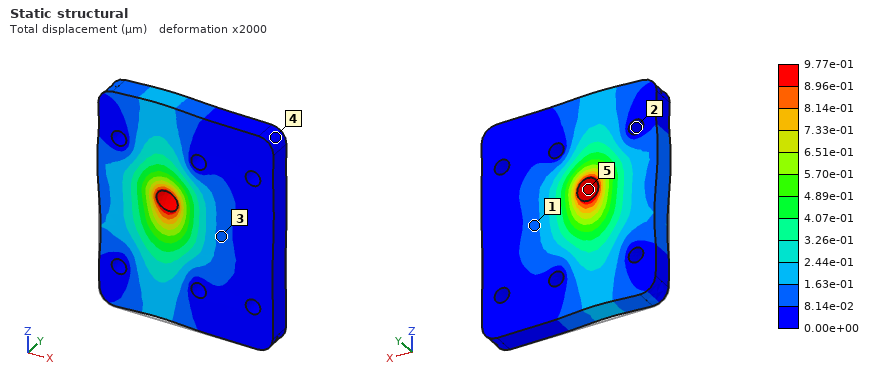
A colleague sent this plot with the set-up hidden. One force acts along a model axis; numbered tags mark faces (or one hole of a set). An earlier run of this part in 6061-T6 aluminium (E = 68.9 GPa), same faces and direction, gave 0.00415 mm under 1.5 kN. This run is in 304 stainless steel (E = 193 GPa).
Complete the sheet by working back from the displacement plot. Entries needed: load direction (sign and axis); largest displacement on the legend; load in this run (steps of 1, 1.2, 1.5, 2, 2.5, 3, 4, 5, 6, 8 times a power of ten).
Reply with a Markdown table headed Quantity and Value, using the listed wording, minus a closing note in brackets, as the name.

| Quantity | Value |
|---|---|
| load direction | +Z |
| largest displacement on the legend | 9.77e-01 µm |
| load in this run | 1 kN |
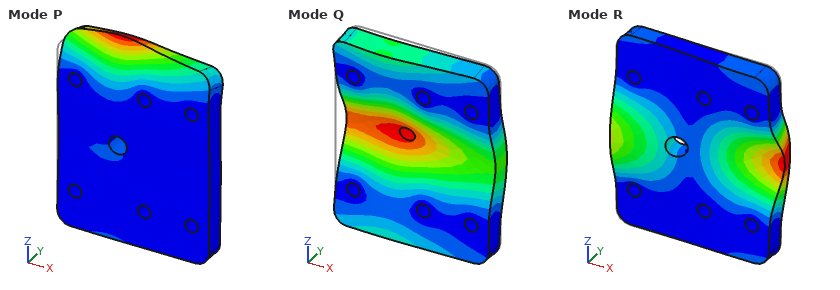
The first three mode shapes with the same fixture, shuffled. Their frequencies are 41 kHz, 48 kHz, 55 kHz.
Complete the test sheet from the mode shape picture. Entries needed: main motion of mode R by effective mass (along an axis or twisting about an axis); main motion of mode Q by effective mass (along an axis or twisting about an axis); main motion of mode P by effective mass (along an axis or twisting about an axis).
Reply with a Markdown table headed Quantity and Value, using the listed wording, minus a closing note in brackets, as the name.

| Quantity | Value |
|---|---|
| main motion of mode R by effective mass | twisting about Z |
| main motion of mode Q by effective mass | along Y |
| main motion of mode P by effective mass | along Y |
